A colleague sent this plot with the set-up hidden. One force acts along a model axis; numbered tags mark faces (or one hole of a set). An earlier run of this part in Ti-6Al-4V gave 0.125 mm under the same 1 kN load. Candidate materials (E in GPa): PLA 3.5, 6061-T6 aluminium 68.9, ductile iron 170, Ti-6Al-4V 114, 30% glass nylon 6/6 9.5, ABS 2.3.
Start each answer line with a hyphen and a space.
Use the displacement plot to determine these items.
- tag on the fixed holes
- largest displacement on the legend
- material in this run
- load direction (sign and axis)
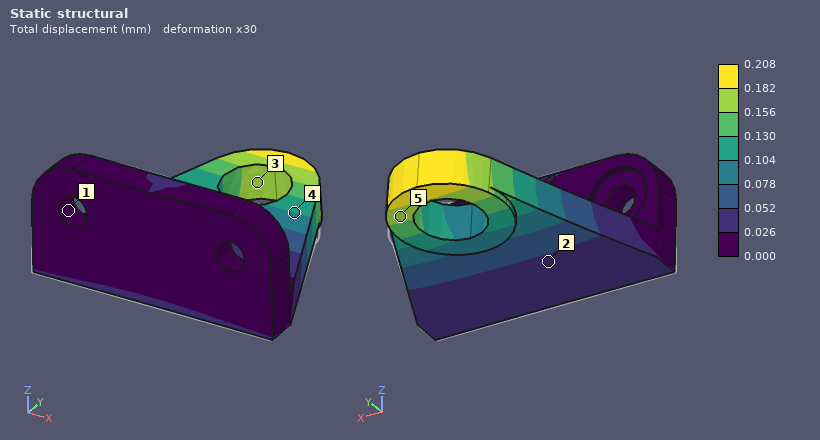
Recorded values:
- 1
- 0.208 mm
- 6061-T6 aluminium
- +Z
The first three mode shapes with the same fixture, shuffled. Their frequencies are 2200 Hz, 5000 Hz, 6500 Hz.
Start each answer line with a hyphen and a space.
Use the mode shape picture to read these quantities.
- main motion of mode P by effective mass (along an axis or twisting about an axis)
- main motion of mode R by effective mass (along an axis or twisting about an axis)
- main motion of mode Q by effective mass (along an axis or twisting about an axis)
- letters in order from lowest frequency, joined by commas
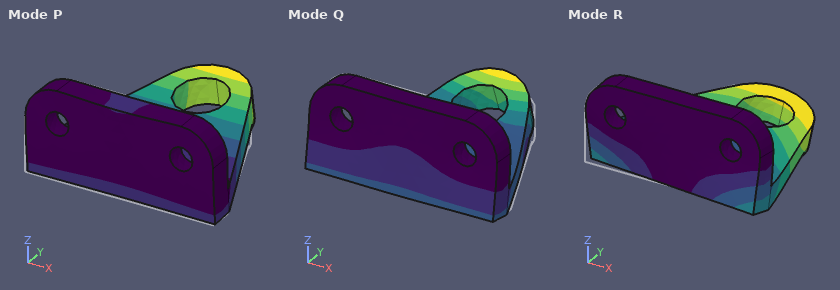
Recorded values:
- along Z
- along X
- along Y
- P, R, Q
